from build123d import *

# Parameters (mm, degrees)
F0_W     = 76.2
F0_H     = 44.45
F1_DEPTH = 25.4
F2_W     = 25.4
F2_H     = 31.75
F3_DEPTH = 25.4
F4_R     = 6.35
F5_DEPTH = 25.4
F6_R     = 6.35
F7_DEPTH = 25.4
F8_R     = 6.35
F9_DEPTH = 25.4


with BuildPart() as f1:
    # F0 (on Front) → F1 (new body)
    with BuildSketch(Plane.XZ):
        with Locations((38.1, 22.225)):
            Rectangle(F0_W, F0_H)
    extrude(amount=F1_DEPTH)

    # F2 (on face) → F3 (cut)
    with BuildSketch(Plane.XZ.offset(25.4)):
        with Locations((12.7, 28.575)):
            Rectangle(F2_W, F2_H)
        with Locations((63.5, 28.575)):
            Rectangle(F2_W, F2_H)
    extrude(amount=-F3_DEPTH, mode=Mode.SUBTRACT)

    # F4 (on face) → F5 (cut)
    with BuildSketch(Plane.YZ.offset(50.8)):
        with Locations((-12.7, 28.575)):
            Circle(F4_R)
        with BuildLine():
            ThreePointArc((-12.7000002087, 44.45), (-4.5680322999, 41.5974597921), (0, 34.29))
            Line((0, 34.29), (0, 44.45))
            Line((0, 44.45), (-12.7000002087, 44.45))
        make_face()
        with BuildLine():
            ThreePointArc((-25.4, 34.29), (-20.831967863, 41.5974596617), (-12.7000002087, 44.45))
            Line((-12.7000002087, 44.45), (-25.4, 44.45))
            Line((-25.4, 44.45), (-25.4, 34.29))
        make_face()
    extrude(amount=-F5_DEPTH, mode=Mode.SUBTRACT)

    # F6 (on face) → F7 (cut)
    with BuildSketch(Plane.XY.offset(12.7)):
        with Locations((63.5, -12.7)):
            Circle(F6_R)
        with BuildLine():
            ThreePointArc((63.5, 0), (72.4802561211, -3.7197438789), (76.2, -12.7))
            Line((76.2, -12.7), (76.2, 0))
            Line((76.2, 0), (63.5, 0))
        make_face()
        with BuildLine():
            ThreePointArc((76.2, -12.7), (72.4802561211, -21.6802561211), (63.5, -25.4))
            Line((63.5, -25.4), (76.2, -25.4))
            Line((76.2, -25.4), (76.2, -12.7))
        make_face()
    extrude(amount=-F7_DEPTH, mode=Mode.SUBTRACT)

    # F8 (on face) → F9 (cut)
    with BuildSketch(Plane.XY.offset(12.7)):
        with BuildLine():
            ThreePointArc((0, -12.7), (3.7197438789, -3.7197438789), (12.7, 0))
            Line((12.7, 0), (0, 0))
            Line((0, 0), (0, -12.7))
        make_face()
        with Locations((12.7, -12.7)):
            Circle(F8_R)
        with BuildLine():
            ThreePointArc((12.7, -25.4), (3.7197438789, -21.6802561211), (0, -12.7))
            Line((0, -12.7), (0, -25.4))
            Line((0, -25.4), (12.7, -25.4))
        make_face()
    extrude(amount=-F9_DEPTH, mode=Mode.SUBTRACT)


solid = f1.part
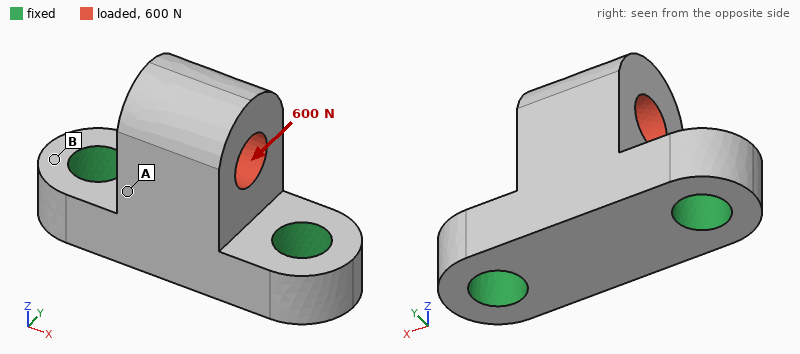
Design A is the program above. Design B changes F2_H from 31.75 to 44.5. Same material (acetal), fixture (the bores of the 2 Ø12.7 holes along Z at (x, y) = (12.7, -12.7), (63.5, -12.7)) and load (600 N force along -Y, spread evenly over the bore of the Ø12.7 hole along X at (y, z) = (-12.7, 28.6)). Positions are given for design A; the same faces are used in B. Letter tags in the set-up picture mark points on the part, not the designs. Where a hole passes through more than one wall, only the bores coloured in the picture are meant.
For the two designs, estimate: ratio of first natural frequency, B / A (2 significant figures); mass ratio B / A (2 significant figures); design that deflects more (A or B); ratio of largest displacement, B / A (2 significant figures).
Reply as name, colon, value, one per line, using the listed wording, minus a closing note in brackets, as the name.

ratio of first natural frequency, B / A: 0.51
mass ratio B / A: 0.84
design that deflects more: B
ratio of largest displacement, B / A: 3.8
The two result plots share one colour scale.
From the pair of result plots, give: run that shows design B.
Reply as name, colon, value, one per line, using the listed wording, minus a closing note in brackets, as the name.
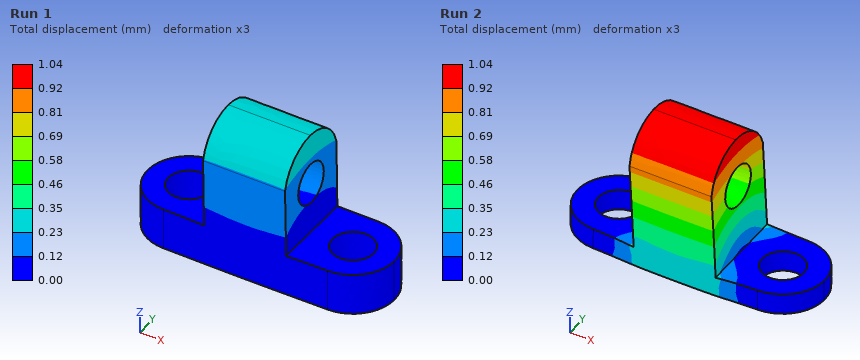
run that shows design B: Run 2
